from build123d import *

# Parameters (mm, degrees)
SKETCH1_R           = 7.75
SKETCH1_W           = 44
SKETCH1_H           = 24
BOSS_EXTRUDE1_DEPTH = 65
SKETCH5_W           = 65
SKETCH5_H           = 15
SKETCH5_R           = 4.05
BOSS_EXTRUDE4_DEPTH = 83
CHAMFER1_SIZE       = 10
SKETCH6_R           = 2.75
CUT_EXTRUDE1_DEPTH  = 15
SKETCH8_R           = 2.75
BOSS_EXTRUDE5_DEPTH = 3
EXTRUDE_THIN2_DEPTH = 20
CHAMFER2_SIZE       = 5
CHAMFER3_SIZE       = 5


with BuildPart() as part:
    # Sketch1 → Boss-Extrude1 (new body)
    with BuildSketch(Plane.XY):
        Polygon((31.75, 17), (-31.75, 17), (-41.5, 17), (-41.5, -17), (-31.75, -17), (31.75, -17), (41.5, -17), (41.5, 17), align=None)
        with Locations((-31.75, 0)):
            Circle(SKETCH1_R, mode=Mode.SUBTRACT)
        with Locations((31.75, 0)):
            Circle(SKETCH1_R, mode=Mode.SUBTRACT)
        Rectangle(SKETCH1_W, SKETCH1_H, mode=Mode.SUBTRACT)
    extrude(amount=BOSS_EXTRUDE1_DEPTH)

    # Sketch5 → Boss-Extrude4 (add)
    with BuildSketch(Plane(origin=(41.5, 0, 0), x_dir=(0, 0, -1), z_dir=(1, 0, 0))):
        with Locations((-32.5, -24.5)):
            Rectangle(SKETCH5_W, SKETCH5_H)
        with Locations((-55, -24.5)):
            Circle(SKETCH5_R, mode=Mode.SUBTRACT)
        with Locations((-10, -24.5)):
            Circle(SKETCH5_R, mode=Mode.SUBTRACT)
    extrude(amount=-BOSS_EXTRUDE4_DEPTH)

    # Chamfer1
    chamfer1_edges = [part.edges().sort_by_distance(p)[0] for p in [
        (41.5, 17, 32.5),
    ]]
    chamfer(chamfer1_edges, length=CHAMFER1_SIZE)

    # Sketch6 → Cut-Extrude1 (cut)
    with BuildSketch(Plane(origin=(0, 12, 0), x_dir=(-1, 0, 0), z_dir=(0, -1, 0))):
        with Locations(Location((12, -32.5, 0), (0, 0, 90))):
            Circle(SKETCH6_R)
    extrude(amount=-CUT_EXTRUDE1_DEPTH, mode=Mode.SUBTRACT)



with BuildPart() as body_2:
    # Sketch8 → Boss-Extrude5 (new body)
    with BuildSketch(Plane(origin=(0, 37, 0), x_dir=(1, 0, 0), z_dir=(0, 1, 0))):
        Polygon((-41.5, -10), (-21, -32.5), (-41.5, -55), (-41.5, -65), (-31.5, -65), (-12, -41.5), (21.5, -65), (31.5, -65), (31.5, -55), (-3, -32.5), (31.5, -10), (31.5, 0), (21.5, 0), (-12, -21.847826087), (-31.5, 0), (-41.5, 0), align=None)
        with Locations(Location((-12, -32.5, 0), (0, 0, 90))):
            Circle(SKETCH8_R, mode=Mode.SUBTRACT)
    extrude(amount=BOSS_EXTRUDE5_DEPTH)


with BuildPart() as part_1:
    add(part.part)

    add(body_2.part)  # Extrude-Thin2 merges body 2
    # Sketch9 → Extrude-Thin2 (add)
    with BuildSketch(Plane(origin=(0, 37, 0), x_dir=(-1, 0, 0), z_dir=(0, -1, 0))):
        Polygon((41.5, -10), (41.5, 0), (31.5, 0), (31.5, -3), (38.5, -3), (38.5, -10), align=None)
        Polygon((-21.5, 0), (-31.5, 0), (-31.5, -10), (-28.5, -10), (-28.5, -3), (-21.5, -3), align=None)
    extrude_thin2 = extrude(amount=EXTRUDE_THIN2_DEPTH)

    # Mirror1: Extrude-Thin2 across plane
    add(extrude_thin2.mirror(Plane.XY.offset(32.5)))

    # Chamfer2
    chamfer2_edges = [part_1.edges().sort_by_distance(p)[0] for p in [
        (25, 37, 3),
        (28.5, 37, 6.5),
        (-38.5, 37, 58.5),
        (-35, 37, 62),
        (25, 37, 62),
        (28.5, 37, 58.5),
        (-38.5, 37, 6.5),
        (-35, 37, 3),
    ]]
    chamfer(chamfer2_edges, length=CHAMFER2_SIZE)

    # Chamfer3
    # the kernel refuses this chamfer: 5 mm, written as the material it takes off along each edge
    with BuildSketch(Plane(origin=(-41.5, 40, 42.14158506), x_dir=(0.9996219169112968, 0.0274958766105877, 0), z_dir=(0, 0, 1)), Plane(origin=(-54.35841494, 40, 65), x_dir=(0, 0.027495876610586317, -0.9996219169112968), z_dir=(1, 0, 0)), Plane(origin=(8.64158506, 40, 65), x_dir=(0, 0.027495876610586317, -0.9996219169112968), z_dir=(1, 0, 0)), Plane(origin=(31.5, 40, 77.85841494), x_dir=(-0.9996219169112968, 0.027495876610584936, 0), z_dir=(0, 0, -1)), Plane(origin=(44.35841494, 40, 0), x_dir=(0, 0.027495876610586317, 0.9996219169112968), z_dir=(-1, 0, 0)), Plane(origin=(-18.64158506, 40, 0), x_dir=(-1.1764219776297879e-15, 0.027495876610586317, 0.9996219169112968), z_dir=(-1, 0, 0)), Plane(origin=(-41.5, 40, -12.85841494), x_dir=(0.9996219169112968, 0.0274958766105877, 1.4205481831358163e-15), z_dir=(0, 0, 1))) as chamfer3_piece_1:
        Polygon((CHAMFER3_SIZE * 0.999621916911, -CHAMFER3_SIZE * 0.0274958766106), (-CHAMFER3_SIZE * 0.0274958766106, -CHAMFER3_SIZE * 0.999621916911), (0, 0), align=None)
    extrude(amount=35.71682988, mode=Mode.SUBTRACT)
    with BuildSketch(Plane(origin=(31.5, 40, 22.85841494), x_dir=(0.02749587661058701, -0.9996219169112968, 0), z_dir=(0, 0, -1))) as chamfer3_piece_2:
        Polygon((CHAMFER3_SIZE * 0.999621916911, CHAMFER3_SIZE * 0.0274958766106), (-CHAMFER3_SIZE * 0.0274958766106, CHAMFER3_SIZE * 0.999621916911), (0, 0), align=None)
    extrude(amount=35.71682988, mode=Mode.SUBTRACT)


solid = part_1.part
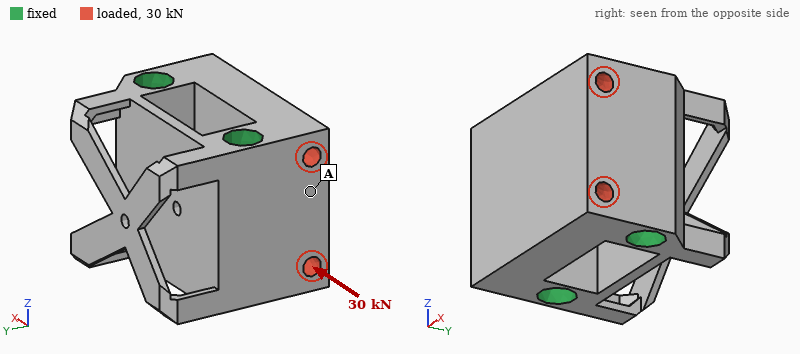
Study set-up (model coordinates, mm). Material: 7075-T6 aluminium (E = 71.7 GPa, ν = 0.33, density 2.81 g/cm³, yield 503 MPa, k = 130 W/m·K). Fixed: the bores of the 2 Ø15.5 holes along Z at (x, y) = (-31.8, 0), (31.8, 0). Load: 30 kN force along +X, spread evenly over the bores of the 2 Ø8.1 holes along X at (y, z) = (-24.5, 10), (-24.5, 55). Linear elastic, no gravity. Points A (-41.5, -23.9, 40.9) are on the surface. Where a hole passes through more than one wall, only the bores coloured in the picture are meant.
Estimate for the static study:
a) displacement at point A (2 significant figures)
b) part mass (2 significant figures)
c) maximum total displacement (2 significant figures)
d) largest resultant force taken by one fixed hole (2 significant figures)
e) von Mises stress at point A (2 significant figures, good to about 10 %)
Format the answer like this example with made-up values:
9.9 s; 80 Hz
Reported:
9.3 µm; 480 g; 15 µm; 16 kN; 7.2 MPa
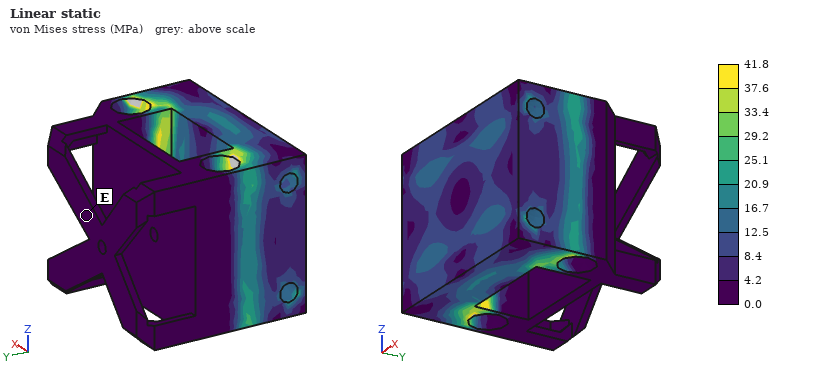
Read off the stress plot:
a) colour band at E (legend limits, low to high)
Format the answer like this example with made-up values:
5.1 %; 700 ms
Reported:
0.0 to 4.2 MPa
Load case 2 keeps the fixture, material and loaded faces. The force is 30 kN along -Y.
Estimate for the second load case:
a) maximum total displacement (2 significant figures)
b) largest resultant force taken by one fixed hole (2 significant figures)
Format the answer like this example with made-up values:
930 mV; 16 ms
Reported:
15 µm; 16 kN
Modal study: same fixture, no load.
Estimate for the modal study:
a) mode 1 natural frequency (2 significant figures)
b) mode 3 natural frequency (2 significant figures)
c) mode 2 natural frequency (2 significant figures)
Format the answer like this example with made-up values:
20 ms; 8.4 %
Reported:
2700 Hz; 3900 Hz; 3800 Hz
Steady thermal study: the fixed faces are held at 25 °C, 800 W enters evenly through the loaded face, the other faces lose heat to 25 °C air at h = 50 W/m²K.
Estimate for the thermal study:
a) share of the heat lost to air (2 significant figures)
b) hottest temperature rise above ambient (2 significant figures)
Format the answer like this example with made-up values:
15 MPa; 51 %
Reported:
3.6 %; 63 K
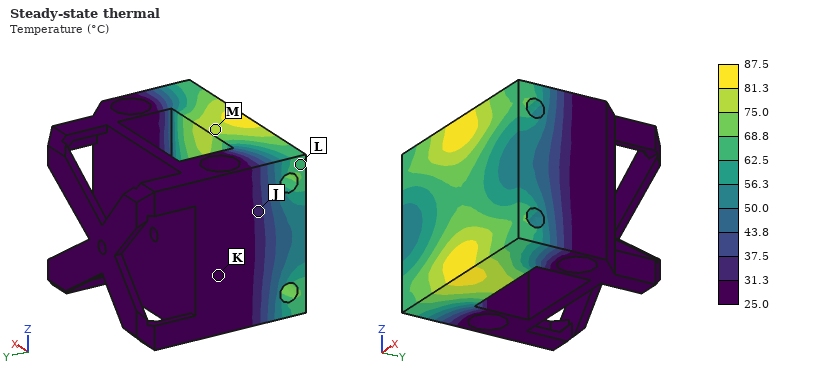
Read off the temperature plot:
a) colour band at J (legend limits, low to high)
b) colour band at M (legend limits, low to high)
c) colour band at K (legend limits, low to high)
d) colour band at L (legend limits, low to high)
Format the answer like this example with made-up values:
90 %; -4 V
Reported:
31.3 to 37.5 °C; 75.0 to 81.3 °C; 25.0 to 31.3 °C; 62.5 to 68.8 °C
